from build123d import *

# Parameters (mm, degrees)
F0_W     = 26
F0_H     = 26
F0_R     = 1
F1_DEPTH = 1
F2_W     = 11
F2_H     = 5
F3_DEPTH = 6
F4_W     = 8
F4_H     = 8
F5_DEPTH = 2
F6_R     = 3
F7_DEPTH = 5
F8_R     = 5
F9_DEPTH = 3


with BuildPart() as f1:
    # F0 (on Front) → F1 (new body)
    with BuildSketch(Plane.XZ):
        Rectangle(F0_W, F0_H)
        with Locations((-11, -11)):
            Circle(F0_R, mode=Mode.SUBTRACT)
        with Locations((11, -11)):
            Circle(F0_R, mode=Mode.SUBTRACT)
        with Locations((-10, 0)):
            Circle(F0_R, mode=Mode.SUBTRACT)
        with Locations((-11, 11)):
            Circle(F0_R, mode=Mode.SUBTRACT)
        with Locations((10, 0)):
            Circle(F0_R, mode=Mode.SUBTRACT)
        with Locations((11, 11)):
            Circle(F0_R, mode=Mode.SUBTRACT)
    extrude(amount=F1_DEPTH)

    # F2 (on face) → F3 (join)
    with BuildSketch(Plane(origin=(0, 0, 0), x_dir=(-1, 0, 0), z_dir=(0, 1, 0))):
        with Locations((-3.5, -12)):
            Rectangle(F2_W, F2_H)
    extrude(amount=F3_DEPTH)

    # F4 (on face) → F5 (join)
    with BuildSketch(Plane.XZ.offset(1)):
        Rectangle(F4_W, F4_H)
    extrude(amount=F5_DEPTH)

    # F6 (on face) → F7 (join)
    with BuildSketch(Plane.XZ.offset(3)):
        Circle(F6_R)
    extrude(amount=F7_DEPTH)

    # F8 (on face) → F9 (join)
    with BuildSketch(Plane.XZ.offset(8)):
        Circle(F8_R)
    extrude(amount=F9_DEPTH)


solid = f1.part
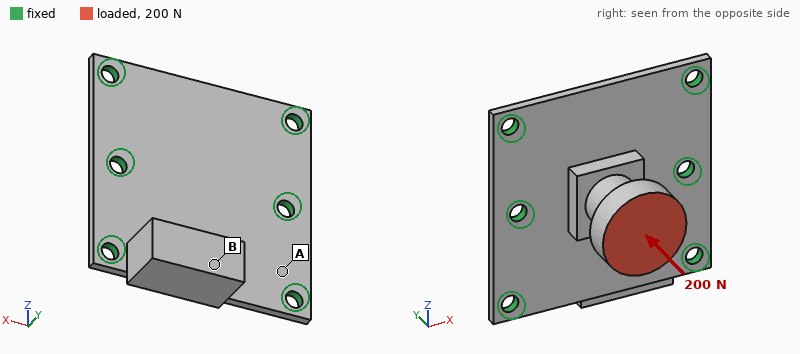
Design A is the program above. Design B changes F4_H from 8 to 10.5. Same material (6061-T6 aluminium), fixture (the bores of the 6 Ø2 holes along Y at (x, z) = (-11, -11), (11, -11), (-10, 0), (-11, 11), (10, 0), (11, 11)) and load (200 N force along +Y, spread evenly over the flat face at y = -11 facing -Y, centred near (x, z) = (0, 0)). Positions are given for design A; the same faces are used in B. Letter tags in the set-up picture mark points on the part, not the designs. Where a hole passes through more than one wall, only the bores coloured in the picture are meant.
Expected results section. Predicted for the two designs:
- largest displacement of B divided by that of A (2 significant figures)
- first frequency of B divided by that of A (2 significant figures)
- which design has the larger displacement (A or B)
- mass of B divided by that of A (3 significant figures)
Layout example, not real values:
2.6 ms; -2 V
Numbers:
0.92; 1.1; A; 1.03
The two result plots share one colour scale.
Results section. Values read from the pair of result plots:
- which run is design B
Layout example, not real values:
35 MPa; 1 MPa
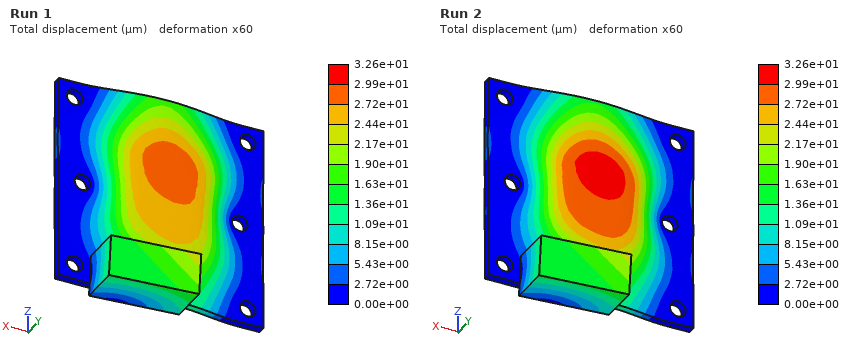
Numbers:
Run 1
